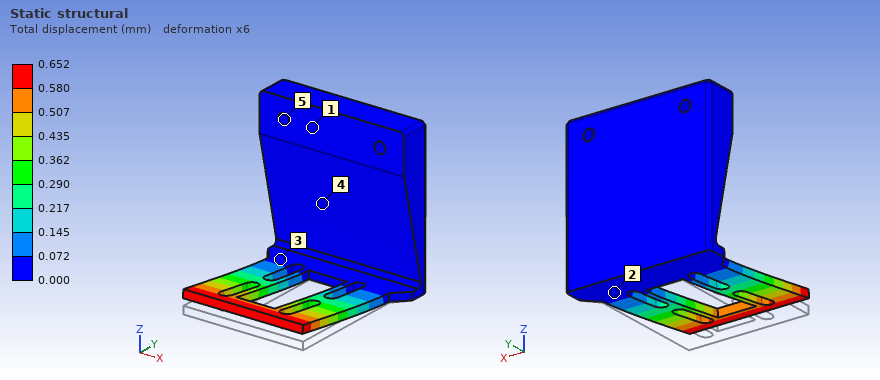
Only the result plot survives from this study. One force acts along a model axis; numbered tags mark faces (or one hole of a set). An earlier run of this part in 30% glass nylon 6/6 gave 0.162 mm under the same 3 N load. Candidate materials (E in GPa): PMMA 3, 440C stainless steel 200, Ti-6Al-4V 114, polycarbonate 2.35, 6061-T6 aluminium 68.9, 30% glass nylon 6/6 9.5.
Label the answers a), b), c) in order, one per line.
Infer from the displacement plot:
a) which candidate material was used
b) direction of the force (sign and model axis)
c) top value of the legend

a) polycarbonate
b) +Z
c) 0.652 mm
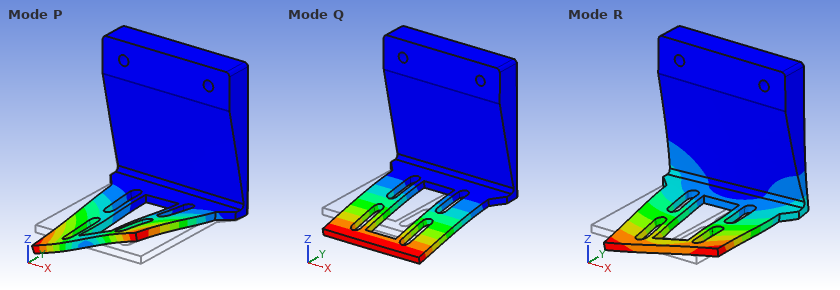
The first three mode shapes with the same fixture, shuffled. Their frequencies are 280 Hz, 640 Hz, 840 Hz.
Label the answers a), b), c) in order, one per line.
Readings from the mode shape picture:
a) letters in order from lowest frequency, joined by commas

a) Q, P, R
